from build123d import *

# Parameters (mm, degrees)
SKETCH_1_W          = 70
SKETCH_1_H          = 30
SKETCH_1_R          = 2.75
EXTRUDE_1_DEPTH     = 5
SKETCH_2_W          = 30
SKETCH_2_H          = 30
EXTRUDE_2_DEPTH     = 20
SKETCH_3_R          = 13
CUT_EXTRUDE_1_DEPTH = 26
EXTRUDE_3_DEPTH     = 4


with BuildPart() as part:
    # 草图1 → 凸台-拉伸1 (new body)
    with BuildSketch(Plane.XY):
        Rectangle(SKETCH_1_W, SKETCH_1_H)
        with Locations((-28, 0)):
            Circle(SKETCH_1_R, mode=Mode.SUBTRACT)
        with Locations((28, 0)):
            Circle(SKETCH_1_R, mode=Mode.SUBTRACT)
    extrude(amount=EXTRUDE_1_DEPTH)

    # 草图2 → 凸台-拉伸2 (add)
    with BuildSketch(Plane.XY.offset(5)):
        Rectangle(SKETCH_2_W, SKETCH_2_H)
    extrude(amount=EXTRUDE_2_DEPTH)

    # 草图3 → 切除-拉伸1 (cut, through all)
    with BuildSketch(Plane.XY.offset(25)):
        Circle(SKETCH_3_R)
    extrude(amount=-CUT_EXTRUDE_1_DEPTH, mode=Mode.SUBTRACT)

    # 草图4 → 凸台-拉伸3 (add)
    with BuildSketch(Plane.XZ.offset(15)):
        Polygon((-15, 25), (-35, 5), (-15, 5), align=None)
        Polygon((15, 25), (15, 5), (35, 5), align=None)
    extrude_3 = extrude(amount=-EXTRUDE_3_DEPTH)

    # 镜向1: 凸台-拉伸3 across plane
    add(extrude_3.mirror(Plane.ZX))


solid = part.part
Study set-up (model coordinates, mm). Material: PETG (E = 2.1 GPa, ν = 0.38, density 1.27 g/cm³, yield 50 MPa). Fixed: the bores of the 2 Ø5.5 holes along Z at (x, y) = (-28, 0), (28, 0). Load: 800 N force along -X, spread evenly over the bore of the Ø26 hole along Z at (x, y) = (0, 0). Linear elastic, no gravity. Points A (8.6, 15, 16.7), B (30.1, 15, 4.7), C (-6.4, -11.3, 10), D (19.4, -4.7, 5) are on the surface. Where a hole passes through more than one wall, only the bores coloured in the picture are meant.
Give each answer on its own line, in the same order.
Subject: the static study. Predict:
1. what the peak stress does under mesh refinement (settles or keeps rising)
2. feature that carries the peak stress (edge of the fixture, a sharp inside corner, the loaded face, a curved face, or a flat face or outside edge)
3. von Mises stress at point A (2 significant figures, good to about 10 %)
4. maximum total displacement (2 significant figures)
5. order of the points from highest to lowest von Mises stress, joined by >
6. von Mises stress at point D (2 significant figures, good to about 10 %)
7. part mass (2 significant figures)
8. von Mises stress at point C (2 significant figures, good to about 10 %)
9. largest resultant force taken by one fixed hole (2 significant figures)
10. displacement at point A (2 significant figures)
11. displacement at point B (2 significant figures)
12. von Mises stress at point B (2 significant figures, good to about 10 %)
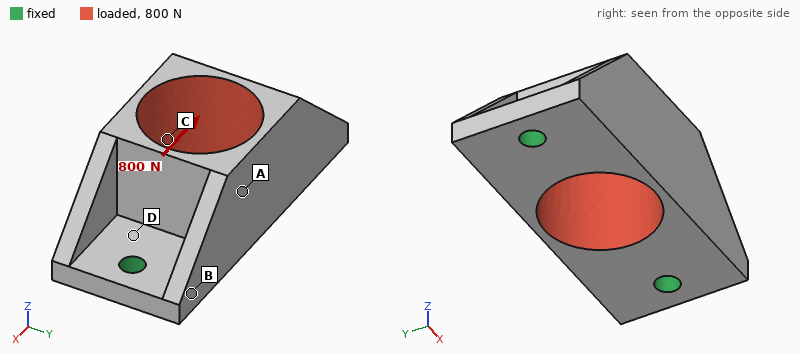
keeps rising
edge of the fixture
2.0 MPa
0.17 mm
D > C > A > B
6.1 MPa
23 g
3.1 MPa
430 N
0.078 mm
0.079 mm
1.0 MPa
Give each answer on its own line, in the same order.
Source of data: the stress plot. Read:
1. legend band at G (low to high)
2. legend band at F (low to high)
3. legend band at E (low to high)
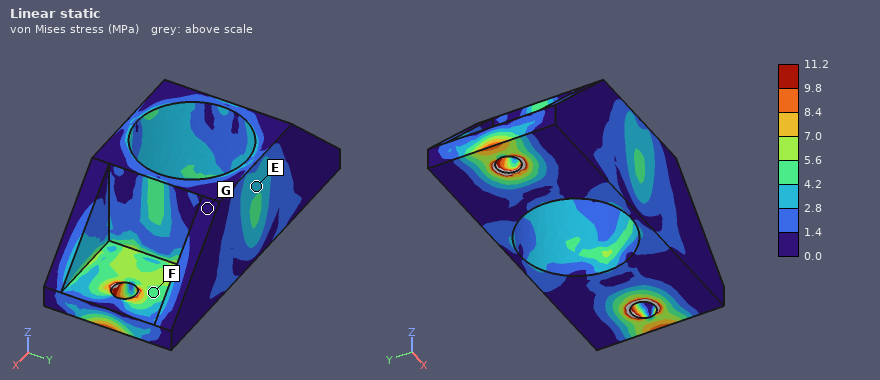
0.0 to 1.4 MPa
4.2 to 5.6 MPa
2.8 to 4.2 MPa
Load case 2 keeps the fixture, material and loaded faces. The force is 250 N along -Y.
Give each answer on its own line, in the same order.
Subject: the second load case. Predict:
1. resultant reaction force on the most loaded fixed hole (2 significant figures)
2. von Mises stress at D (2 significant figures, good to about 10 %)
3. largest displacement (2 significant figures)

130 N
4.2 MPa
0.35 mm
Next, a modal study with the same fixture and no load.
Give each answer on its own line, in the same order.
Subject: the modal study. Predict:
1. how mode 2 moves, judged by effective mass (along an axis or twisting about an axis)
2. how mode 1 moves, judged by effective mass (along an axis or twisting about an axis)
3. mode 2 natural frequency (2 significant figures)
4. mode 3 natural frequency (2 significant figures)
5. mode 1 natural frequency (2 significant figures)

along Z
along Y
2400 Hz
2600 Hz
1200 Hz
